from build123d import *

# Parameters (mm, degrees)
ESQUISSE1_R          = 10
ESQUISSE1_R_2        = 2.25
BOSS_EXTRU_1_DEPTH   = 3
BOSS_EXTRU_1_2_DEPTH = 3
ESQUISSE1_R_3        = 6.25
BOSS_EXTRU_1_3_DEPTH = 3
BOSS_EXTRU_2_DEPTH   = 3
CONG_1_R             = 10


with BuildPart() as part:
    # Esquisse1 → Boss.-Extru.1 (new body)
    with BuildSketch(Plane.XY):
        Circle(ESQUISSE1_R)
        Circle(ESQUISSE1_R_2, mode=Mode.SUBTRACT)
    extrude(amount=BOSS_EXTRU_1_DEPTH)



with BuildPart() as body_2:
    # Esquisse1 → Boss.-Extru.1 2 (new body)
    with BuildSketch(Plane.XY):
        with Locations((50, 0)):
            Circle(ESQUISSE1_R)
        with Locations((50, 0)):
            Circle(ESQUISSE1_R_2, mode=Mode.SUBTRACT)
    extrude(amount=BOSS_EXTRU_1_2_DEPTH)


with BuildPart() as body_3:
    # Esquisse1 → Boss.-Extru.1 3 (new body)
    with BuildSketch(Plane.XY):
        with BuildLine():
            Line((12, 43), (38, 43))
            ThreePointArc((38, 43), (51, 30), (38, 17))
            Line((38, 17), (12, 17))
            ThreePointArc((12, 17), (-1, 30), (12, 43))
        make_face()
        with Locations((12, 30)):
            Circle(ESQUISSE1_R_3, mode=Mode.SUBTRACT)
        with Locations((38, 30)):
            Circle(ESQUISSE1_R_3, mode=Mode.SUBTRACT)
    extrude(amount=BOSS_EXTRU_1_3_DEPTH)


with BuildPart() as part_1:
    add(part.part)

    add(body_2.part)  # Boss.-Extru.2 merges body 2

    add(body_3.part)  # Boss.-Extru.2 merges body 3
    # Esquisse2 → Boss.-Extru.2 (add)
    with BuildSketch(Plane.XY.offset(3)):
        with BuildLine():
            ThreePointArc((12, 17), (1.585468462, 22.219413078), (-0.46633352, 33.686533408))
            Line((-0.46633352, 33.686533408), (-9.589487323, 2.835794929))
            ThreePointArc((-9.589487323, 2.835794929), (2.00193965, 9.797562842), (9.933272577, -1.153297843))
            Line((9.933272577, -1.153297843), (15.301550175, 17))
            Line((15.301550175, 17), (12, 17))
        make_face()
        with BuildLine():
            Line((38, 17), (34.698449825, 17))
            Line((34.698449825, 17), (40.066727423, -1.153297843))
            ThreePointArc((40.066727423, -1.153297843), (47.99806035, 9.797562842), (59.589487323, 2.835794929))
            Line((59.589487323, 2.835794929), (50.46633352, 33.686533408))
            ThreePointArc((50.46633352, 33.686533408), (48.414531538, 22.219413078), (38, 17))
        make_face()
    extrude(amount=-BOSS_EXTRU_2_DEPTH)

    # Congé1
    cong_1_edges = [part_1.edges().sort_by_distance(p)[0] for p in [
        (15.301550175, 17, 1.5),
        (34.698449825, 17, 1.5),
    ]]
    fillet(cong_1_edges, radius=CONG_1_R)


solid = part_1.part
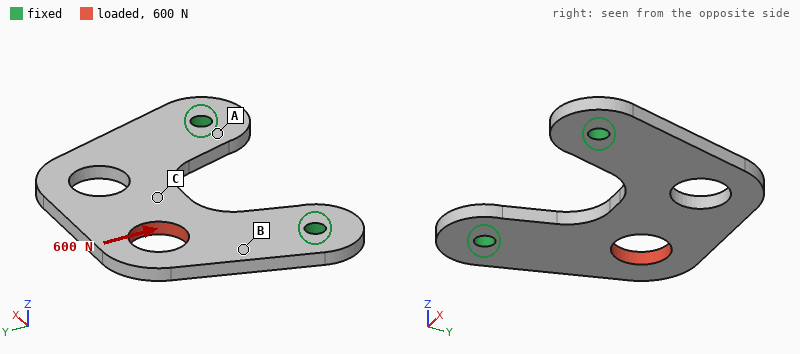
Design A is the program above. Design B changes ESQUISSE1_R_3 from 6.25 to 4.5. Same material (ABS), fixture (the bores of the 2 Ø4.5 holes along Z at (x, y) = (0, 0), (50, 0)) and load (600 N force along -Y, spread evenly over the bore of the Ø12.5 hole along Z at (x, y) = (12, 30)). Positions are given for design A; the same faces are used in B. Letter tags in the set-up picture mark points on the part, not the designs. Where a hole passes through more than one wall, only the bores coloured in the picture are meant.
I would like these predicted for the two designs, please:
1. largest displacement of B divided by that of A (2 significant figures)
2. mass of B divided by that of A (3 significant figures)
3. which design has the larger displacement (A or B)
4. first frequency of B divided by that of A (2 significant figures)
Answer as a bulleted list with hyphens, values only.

- 0.91
- 1.06
- A
- 0.96
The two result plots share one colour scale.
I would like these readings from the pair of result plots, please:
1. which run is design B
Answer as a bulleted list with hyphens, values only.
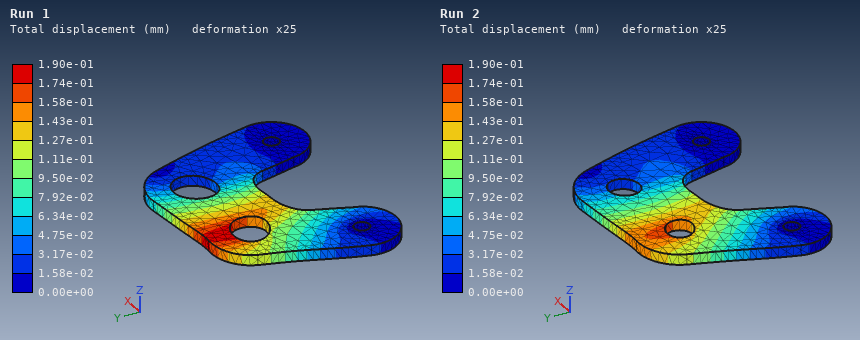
- Run 2
